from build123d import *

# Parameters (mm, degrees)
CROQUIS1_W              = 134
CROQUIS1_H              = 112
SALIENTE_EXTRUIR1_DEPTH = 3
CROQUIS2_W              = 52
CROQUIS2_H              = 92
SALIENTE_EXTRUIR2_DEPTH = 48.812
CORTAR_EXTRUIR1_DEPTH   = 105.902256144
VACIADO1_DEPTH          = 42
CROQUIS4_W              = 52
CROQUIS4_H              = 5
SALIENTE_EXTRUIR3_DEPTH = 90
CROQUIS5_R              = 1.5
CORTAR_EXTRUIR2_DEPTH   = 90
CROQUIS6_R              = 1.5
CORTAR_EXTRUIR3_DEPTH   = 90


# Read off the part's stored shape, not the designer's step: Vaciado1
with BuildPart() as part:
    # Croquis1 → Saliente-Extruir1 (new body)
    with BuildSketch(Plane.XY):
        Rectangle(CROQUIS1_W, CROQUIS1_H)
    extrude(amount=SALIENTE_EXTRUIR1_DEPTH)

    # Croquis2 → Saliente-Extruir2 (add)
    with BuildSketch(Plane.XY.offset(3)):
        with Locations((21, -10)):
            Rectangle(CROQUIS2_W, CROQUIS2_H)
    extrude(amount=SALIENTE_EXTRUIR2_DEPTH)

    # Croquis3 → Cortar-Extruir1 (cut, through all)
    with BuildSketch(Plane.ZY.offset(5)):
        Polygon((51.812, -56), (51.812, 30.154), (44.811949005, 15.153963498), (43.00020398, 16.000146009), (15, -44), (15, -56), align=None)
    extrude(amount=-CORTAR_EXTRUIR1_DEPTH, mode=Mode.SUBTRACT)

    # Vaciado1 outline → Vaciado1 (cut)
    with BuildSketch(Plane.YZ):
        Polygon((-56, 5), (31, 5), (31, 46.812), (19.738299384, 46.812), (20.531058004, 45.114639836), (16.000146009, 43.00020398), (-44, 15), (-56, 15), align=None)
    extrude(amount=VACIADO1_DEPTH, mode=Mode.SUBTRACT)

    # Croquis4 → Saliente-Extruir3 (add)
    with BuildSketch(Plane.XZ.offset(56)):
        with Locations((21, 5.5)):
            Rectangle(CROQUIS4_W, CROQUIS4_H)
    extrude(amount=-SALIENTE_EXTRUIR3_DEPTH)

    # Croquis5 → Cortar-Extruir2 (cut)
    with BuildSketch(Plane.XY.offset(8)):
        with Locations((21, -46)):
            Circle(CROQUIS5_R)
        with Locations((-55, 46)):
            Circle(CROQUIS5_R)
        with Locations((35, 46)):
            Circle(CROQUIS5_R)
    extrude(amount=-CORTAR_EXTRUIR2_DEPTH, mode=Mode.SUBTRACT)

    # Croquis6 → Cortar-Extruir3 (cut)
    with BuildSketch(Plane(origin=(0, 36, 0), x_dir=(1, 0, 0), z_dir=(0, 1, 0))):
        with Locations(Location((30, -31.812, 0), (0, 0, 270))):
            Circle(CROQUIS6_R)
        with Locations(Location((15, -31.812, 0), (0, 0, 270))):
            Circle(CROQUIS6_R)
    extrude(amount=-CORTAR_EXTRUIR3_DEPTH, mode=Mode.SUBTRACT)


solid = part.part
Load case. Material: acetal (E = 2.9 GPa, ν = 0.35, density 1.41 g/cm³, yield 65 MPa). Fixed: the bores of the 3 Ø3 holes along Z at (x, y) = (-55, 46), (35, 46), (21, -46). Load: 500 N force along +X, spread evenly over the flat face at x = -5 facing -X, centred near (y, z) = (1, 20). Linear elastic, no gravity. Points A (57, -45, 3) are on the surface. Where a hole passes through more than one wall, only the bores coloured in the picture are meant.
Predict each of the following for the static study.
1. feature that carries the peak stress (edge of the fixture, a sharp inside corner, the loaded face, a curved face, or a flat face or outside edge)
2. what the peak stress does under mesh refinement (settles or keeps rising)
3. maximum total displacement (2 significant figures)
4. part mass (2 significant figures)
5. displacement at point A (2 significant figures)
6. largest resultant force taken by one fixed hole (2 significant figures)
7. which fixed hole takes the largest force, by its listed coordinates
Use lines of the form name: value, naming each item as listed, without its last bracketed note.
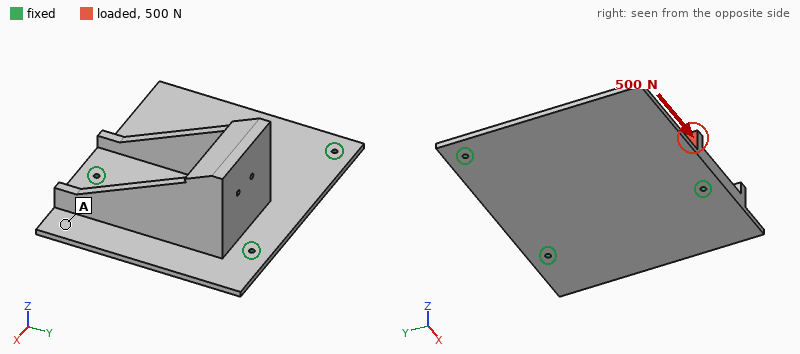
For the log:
feature that carries the peak stress: edge of the fixture
what the peak stress does under mesh refinement: keeps rising
maximum total displacement: 1.7 mm
part mass: 140 g
displacement at point A: 0.44 mm
largest resultant force taken by one fixed hole: 360 N
which fixed hole takes the largest force, by its listed coordinates: (21, -46)
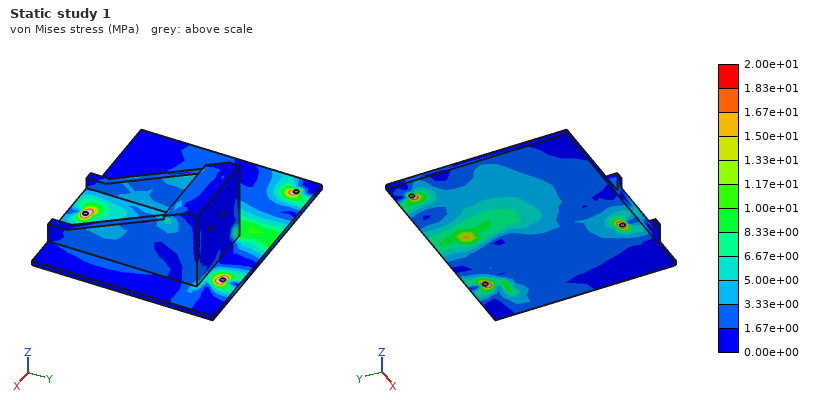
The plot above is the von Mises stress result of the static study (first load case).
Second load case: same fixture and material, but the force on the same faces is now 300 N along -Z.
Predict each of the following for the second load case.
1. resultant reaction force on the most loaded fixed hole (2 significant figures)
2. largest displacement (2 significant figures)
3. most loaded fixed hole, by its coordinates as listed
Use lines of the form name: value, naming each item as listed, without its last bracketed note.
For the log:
resultant reaction force on the most loaded fixed hole: 220 N
largest displacement: 1.7 mm
most loaded fixed hole, by its coordinates as listed: (21, -46)
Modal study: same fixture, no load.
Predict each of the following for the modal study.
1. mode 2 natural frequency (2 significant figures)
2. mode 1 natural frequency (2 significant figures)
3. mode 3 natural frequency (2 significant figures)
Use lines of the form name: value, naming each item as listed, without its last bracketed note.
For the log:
mode 2 natural frequency: 330 Hz
mode 1 natural frequency: 220 Hz
mode 3 natural frequency: 590 Hz
